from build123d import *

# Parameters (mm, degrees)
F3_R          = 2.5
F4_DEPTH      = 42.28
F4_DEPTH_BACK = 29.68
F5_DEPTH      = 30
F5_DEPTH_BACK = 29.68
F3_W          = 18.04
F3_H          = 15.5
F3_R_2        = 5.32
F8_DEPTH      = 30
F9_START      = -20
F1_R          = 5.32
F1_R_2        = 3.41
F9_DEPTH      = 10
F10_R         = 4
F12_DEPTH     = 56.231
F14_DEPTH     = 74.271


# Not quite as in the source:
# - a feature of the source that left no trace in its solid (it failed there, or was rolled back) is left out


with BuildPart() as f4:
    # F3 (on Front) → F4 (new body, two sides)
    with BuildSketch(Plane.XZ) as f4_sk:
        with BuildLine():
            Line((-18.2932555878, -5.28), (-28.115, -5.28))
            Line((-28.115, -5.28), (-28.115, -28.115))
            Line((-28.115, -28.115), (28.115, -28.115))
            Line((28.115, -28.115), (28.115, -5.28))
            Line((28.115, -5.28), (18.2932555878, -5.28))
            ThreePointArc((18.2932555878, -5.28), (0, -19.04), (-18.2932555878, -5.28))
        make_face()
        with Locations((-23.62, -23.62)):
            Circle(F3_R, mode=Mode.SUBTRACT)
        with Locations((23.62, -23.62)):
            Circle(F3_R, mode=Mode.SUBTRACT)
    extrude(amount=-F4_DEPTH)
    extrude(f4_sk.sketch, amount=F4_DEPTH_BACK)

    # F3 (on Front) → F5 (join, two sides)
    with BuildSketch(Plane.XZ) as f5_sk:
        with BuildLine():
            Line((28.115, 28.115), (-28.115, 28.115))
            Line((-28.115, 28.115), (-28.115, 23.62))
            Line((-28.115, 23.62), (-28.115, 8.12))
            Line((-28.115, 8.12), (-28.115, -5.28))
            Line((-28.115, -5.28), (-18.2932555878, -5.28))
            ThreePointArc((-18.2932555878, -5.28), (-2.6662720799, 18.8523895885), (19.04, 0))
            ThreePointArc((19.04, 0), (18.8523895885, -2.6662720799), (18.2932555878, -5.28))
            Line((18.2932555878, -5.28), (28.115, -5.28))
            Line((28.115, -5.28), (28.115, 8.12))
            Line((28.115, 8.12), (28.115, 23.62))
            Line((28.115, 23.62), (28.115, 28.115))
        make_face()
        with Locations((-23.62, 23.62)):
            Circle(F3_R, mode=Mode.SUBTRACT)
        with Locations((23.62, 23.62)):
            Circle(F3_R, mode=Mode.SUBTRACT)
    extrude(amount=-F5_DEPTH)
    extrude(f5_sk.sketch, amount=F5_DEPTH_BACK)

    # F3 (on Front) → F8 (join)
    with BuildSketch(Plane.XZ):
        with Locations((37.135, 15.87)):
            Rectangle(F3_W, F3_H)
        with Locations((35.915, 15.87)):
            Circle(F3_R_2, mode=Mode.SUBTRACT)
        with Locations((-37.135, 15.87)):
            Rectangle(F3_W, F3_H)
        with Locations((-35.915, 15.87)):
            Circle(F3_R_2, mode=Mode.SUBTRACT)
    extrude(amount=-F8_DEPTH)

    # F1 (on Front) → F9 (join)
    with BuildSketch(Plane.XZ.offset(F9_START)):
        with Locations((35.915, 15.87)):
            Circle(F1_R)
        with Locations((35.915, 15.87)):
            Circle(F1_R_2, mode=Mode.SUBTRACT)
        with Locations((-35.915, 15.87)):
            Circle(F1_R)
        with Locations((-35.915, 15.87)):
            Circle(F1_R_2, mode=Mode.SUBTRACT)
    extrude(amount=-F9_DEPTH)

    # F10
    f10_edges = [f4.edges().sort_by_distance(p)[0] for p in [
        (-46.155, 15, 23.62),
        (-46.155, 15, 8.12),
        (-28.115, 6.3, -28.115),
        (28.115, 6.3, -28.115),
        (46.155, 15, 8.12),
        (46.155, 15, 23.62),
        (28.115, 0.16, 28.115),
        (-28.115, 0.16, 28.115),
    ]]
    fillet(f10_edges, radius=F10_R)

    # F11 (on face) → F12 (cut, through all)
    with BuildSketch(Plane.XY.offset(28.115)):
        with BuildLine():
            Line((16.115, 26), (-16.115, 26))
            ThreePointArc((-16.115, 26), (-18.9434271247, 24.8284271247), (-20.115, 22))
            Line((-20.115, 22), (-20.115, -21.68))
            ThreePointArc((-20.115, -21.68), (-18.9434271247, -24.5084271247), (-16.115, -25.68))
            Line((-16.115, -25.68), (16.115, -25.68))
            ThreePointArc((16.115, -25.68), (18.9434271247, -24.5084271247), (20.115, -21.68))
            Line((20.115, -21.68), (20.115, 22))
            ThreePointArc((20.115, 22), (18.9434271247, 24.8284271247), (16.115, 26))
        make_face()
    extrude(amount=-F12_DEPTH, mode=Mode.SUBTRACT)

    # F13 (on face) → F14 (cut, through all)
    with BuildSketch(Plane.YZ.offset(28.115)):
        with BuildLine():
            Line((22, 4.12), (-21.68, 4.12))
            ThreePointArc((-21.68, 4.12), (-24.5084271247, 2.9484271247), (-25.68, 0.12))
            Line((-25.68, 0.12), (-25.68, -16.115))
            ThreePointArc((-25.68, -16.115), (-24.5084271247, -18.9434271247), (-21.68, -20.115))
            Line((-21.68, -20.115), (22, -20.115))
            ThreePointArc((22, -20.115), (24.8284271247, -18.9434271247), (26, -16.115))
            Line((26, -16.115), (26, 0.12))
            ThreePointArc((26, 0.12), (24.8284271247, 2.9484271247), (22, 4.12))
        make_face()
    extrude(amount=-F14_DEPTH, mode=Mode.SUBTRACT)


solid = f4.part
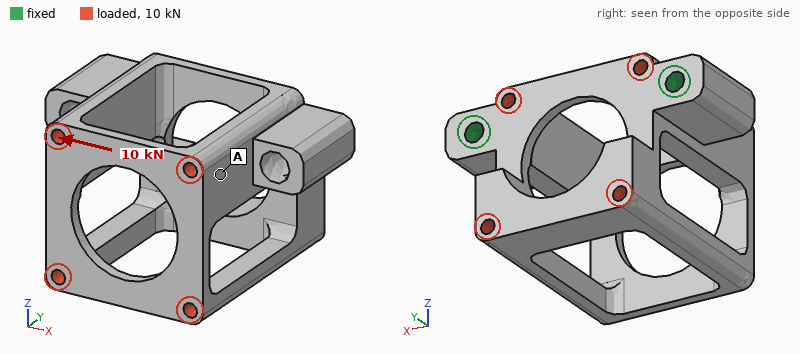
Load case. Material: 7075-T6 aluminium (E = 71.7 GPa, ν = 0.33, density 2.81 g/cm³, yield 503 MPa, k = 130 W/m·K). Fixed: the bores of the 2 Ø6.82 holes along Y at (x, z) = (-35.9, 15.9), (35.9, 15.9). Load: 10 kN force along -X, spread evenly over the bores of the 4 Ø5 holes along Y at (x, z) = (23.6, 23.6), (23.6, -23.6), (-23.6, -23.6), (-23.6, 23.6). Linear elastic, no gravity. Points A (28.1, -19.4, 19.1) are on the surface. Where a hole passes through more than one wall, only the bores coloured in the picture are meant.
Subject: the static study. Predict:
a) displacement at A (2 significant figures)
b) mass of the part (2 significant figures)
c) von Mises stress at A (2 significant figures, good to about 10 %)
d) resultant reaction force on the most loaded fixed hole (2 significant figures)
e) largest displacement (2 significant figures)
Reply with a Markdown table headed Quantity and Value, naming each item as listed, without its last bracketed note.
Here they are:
| Quantity | Value |
|---|---|
| displacement at A | 0.22 mm |
| mass of the part | 170 g |
| von Mises stress at A | 39 MPa |
| resultant reaction force on the most loaded fixed hole | 5.8 kN |
| largest displacement | 0.49 mm |
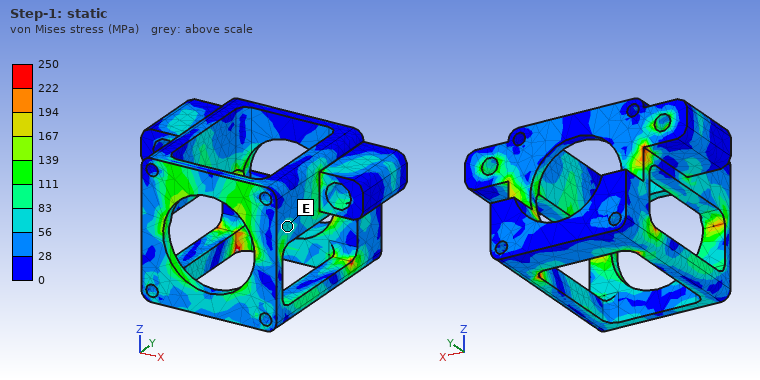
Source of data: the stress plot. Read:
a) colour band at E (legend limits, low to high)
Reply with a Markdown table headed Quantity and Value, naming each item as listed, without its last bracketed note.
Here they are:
| Quantity | Value |
|---|---|
| colour band at E | 56 to 83 MPa |
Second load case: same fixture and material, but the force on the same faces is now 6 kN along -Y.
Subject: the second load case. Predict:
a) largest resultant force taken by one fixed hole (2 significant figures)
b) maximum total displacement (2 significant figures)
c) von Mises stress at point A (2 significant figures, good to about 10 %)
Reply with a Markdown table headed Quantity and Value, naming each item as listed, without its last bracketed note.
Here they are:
| Quantity | Value |
|---|---|
| largest resultant force taken by one fixed hole | 3.0 kN |
| maximum total displacement | 0.54 mm |
| von Mises stress at point A | 20 MPa |
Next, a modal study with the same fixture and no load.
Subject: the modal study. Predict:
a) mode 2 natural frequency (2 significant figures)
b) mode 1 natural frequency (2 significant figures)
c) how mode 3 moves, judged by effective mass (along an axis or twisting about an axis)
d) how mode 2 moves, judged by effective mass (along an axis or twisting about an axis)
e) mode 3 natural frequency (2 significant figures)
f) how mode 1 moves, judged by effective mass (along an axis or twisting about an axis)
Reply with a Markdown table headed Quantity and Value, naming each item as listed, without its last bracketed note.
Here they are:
| Quantity | Value |
|---|---|
| mode 2 natural frequency | 2700 Hz |
| mode 1 natural frequency | 1700 Hz |
| how mode 3 moves, judged by effective mass | along Z |
| how mode 2 moves, judged by effective mass | along X |
| mode 3 natural frequency | 3500 Hz |
| how mode 1 moves, judged by effective mass | along Y |
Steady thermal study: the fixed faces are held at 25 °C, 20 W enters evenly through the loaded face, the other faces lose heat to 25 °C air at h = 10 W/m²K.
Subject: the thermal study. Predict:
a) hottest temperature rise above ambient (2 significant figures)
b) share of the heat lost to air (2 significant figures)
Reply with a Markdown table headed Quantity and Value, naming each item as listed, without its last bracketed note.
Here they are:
| Quantity | Value |
|---|---|
| hottest temperature rise above ambient | 20 K |
| share of the heat lost to air | 11 % |
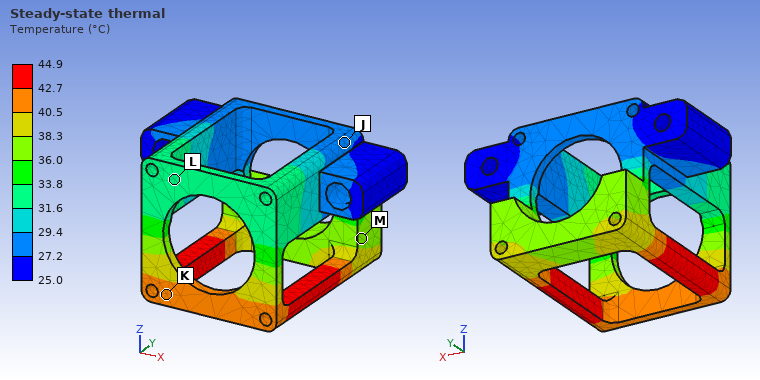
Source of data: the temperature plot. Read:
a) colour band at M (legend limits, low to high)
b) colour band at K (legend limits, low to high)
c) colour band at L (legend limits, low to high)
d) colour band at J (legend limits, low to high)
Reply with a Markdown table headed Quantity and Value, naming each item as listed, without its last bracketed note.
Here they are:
| Quantity | Value |
|---|---|
| colour band at M | 36.0 to 38.3 °C |
| colour band at K | 40.5 to 42.7 °C |
| colour band at L | 31.6 to 33.8 °C |
| colour band at J | 27.2 to 29.4 °C |
